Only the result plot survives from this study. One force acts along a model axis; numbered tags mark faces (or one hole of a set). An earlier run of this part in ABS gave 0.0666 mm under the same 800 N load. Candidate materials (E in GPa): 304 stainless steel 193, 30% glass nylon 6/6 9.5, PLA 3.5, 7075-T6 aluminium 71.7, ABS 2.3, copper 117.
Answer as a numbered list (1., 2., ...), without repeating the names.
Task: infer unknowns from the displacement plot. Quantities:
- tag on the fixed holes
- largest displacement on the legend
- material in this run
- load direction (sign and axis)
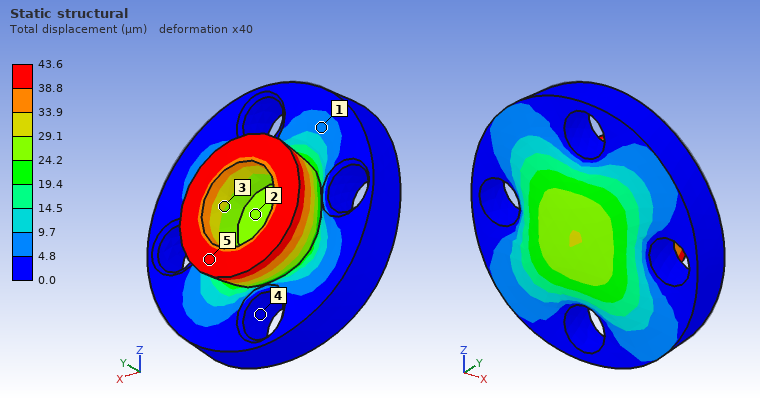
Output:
1. 4
2. 43.6 µm
3. PLA
4. -Y
